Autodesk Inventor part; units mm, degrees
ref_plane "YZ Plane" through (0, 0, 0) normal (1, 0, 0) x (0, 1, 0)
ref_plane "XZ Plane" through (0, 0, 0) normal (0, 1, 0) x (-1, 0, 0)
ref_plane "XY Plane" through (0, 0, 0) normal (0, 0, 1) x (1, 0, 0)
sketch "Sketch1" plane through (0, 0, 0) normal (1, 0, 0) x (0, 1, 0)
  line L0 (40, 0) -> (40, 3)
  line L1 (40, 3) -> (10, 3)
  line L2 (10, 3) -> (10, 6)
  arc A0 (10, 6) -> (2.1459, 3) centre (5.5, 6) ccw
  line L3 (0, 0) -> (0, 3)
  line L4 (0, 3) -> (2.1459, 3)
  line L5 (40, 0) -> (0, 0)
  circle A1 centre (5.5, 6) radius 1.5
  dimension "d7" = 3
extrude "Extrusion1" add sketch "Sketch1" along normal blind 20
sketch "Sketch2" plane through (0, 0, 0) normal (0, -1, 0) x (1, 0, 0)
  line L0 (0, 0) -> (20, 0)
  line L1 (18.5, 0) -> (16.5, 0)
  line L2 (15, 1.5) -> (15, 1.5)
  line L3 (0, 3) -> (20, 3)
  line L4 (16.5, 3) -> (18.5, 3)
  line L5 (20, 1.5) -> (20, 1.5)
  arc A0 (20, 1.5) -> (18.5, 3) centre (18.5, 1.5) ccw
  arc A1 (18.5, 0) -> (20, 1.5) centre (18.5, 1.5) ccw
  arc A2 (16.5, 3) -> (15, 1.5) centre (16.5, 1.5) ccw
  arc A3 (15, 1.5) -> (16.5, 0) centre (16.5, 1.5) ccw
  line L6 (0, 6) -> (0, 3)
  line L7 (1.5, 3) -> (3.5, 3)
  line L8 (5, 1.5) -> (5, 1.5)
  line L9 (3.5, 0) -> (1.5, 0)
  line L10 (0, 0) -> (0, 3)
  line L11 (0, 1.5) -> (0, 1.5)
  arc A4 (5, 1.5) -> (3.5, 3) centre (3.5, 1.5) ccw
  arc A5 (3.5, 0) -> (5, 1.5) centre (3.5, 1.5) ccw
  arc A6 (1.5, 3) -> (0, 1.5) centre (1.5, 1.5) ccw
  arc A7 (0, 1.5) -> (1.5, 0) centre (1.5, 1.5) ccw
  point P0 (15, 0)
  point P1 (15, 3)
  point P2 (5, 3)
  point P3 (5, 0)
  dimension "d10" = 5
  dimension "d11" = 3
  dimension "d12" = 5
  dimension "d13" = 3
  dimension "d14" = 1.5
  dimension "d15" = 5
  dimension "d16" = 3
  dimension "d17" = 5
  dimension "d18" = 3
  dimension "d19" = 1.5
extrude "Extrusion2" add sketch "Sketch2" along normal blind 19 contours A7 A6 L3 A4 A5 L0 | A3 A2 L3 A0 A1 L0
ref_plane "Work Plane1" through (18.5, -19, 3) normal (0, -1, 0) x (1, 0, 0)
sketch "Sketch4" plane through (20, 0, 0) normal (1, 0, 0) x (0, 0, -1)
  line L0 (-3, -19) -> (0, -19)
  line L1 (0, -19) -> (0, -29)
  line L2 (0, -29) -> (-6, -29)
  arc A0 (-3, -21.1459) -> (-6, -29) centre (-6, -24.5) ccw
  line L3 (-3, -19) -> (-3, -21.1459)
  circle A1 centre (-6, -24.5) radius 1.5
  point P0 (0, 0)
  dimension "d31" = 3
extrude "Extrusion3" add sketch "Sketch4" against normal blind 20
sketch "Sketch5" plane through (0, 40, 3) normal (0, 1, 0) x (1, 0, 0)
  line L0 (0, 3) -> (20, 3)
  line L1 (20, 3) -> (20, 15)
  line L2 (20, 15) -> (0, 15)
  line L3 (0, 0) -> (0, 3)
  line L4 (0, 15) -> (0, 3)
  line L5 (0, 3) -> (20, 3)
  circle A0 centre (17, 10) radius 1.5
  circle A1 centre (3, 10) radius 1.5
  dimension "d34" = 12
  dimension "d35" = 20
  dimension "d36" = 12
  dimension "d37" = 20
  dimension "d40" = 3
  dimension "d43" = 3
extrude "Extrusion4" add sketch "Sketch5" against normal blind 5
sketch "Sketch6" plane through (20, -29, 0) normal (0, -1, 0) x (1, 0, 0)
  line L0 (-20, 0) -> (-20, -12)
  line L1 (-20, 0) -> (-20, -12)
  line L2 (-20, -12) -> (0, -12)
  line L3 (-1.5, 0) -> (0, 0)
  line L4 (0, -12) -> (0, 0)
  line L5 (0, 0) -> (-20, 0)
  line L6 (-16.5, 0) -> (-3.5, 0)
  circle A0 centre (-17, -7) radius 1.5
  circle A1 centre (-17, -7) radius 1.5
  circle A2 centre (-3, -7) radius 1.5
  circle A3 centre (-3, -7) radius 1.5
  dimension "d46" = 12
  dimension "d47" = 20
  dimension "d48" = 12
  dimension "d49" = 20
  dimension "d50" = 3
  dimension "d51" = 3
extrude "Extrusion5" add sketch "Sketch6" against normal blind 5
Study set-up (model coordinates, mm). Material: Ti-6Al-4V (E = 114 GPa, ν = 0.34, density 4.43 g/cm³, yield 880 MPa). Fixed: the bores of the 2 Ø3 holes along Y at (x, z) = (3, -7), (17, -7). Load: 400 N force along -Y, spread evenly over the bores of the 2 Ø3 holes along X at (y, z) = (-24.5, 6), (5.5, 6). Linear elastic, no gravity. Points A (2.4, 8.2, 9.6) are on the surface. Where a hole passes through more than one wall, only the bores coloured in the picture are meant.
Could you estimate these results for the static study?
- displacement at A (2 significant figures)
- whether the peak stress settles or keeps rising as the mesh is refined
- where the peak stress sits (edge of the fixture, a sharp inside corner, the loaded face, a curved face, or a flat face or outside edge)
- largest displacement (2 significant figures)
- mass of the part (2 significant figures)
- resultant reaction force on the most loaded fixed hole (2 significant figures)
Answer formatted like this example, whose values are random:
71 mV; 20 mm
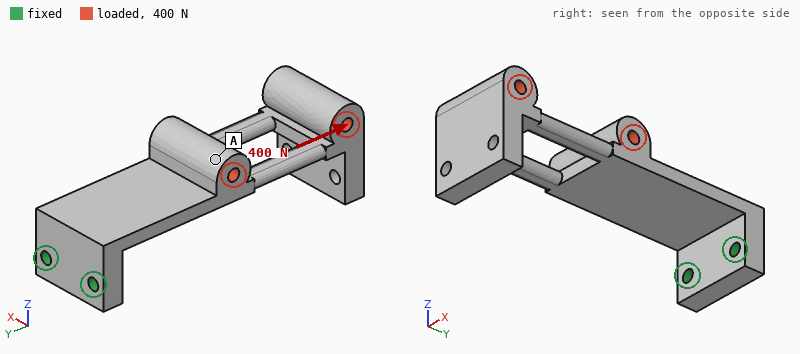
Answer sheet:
0.19 mm; keeps rising; edge of the fixture; 0.83 mm; 34 g; 200 N
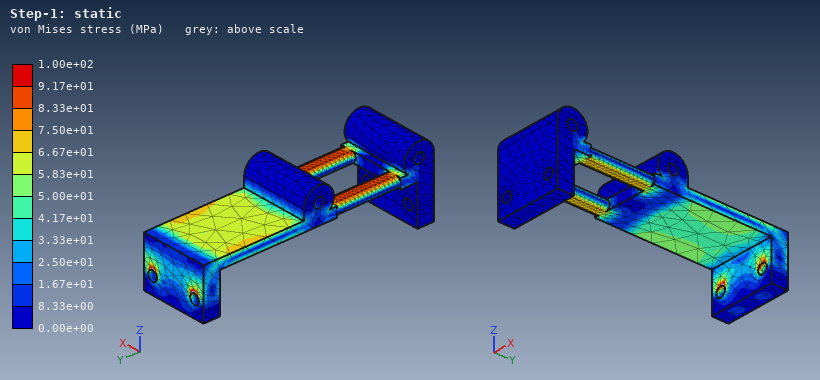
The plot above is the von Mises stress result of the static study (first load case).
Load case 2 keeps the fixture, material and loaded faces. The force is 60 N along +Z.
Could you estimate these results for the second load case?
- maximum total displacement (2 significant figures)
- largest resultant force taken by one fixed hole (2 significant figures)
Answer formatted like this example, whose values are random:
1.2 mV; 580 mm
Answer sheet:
0.75 mm; 51 N
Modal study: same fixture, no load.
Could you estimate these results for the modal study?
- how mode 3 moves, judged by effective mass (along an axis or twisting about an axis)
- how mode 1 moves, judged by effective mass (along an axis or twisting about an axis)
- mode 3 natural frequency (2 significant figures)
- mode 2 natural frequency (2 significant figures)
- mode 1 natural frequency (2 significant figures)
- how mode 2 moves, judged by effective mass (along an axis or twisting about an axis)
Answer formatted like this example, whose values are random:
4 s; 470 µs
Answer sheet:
along Z; along Z; 1800 Hz; 1300 Hz; 320 Hz; along X
